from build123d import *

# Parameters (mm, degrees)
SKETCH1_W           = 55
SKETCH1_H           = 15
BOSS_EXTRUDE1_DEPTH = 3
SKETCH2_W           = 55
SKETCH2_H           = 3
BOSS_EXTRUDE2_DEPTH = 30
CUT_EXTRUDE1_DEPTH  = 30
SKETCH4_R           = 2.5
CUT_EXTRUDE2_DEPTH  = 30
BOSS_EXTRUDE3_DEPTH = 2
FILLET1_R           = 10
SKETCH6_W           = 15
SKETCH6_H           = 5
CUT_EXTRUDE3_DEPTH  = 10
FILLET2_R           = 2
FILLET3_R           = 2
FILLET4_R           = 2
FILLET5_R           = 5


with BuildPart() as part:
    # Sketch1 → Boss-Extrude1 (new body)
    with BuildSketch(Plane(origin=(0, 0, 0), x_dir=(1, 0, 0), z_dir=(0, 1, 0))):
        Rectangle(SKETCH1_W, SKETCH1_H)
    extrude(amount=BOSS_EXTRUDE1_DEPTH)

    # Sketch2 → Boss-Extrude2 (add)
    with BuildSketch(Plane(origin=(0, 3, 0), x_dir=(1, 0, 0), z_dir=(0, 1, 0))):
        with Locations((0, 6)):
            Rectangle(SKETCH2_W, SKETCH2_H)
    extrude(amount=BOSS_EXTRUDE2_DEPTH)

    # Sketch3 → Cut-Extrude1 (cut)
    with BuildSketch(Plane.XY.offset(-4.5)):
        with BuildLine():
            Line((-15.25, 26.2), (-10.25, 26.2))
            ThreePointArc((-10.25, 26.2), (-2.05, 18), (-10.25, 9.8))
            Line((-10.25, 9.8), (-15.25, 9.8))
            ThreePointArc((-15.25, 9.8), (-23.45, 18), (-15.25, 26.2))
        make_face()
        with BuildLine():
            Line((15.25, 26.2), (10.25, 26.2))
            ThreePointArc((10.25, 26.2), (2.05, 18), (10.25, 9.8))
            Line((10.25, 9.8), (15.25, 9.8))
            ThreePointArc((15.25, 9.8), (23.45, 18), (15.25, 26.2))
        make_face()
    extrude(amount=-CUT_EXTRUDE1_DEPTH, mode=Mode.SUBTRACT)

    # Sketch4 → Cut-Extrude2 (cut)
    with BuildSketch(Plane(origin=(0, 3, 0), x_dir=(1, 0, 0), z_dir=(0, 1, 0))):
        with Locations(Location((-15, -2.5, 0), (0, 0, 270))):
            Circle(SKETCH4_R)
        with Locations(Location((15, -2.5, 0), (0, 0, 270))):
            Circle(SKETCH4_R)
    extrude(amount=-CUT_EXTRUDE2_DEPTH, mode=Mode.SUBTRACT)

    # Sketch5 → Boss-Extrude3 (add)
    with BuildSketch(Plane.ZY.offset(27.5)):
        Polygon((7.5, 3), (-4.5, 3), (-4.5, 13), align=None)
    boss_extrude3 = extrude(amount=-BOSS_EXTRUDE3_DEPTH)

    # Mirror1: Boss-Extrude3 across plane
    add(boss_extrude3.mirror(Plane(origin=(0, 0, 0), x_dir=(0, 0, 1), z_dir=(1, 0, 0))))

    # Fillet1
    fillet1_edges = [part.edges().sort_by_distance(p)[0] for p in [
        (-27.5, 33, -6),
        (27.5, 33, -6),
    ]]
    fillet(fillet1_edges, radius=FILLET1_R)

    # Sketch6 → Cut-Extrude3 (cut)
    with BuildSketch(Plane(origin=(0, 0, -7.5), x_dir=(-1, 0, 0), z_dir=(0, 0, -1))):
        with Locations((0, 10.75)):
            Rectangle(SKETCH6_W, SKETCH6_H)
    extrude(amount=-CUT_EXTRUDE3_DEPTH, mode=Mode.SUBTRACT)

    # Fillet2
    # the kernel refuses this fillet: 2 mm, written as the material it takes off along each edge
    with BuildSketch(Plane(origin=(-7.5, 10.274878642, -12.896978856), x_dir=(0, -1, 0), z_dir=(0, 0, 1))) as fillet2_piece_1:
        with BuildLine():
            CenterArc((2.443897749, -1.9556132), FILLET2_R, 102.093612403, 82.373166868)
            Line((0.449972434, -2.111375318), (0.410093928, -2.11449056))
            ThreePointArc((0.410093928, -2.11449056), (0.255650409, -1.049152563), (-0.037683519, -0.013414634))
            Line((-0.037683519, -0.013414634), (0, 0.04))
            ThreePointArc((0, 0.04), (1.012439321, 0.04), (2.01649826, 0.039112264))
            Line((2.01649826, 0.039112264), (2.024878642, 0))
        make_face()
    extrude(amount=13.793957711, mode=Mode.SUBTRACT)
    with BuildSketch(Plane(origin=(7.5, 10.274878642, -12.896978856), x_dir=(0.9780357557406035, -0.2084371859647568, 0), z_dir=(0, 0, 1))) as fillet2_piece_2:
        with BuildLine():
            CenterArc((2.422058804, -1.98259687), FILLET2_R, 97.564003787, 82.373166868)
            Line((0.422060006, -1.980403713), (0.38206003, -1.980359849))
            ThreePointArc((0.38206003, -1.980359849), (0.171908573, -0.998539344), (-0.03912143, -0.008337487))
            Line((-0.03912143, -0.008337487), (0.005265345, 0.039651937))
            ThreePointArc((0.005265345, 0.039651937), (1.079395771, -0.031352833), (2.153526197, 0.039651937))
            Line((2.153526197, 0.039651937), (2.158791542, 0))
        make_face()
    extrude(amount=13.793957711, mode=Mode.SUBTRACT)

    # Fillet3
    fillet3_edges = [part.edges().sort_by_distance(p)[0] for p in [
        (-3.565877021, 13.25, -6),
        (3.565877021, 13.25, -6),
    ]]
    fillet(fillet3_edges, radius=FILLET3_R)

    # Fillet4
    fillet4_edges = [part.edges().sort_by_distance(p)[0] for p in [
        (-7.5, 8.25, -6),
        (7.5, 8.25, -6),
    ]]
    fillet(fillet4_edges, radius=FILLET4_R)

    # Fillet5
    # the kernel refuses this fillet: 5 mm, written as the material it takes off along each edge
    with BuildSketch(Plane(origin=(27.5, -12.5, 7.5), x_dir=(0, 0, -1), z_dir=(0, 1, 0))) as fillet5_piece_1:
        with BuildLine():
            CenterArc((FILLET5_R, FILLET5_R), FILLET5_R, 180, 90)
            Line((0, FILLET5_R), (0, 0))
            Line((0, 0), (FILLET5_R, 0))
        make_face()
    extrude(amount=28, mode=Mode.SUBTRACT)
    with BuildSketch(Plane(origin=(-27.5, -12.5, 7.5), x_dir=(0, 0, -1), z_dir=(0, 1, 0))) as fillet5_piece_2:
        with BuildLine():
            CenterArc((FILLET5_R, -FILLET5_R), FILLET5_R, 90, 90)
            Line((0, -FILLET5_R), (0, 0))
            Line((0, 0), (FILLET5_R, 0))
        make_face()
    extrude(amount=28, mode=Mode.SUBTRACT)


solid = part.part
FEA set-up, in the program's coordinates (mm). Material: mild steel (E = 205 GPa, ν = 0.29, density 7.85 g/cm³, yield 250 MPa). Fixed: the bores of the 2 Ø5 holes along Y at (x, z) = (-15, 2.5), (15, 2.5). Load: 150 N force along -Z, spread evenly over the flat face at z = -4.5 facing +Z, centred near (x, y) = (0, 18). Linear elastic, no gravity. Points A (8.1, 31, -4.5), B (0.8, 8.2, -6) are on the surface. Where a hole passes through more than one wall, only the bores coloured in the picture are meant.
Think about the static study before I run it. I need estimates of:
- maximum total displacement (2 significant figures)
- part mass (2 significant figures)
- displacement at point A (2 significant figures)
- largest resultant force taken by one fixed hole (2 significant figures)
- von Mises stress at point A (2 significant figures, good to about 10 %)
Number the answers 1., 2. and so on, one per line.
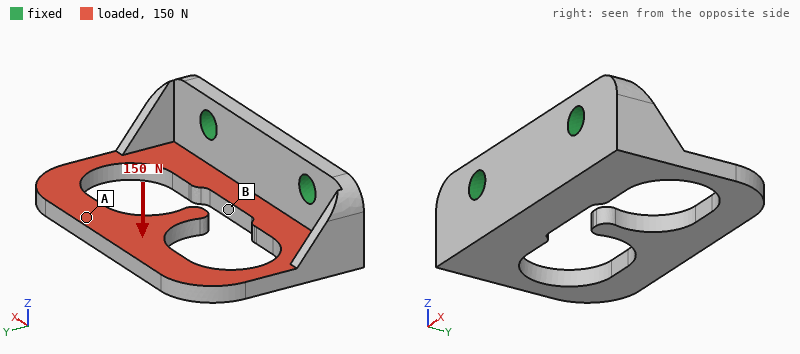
1. 96 µm
2. 43 g
3. 86 µm
4. 75 N
5. 27 MPa
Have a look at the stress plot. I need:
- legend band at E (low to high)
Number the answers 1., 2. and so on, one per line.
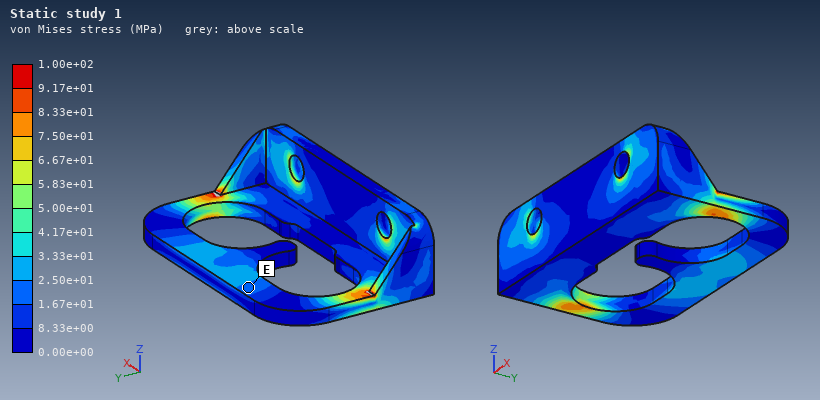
1. 1.67e+01 to 2.50e+01 MPa
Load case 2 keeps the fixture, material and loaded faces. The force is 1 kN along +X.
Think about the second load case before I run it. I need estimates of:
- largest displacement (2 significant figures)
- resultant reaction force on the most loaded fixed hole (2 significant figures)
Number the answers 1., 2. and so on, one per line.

1. 76 µm
2. 710 N
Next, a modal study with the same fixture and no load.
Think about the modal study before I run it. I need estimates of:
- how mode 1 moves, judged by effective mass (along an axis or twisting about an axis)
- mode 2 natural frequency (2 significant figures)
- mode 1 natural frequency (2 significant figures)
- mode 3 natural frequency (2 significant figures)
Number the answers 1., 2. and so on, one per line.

1. along Z
2. 3600 Hz
3. 1600 Hz
4. 4800 Hz
